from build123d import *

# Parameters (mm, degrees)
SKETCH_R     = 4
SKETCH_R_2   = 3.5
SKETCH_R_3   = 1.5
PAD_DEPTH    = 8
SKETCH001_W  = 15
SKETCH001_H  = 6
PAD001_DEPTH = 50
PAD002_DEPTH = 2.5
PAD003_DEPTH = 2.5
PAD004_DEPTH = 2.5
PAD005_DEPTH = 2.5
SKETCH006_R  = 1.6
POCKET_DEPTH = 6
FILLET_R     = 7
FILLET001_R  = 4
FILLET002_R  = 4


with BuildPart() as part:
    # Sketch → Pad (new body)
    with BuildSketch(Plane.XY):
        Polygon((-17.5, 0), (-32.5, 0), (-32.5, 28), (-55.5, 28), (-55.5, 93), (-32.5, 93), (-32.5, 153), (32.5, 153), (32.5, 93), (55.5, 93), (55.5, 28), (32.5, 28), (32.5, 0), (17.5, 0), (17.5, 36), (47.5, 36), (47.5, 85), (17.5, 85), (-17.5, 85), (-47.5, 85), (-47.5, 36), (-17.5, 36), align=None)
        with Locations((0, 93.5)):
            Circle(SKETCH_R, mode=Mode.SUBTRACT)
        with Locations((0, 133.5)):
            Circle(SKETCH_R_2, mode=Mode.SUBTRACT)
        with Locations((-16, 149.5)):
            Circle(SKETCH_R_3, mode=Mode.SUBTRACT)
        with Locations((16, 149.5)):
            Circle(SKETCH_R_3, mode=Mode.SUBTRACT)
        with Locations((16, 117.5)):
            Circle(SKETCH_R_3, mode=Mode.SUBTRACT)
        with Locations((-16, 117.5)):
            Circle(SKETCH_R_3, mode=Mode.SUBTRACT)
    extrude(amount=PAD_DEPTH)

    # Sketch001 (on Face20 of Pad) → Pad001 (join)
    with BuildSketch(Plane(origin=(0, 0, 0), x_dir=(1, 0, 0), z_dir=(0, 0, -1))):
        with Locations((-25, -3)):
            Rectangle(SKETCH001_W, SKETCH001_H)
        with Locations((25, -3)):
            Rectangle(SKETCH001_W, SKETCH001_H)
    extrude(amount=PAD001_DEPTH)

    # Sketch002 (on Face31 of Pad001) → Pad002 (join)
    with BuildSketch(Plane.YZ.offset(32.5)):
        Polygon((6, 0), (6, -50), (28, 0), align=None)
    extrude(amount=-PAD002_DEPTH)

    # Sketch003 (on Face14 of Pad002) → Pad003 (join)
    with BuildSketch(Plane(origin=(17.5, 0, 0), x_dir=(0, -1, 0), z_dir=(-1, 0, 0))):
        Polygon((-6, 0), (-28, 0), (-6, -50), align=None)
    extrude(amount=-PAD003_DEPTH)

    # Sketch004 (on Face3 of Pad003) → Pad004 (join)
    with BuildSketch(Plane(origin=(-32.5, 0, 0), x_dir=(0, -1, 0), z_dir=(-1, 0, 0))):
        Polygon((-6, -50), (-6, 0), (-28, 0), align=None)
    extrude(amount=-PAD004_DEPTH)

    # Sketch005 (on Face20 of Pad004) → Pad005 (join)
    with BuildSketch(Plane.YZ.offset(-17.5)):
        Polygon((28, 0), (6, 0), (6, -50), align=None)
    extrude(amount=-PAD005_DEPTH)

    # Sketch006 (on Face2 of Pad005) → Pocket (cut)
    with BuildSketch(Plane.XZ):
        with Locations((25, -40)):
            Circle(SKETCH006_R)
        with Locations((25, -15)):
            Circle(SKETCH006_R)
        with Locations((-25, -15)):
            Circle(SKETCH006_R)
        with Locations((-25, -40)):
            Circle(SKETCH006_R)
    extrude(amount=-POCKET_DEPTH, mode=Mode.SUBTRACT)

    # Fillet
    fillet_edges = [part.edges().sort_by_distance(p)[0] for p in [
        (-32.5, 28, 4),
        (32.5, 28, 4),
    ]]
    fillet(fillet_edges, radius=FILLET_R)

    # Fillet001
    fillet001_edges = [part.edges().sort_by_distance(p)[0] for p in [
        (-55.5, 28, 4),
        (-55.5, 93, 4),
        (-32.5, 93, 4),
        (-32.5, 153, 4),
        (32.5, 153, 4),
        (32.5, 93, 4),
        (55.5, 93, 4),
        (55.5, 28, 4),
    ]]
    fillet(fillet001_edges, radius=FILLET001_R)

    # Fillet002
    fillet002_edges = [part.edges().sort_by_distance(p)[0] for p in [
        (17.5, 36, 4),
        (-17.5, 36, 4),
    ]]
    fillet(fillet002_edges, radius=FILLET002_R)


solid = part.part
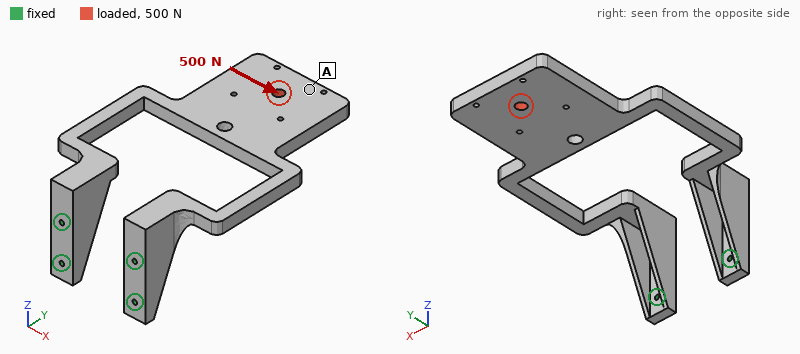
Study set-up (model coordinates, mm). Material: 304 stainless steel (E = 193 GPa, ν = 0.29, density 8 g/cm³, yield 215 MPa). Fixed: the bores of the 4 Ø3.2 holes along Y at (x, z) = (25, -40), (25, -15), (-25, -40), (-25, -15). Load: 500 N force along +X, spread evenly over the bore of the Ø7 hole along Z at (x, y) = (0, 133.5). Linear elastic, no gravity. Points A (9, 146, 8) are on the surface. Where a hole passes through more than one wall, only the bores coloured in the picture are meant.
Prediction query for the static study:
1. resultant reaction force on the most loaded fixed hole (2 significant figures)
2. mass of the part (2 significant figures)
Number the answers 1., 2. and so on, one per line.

1. 760 N
2. 560 g
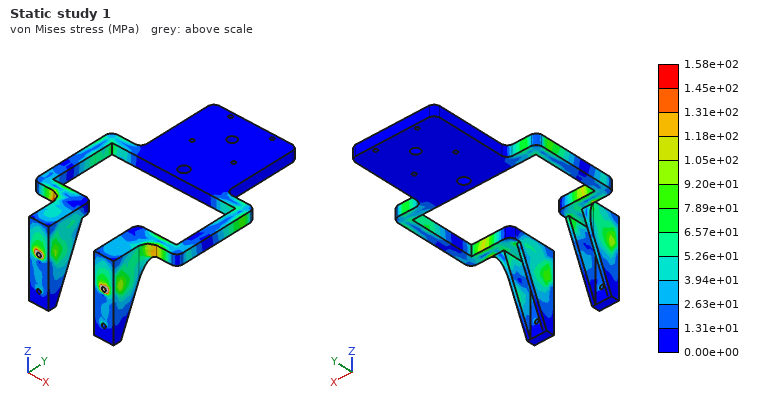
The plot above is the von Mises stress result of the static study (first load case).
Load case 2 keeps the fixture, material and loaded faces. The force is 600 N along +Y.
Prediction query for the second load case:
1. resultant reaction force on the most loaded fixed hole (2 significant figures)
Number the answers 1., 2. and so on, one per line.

1. 490 N
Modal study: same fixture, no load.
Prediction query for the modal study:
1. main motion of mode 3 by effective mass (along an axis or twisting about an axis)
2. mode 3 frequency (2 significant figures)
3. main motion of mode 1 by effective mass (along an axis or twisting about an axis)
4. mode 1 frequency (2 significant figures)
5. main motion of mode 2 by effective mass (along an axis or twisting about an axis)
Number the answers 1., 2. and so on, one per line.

1. twisting about Y
2. 760 Hz
3. along Z
4. 150 Hz
5. along X
